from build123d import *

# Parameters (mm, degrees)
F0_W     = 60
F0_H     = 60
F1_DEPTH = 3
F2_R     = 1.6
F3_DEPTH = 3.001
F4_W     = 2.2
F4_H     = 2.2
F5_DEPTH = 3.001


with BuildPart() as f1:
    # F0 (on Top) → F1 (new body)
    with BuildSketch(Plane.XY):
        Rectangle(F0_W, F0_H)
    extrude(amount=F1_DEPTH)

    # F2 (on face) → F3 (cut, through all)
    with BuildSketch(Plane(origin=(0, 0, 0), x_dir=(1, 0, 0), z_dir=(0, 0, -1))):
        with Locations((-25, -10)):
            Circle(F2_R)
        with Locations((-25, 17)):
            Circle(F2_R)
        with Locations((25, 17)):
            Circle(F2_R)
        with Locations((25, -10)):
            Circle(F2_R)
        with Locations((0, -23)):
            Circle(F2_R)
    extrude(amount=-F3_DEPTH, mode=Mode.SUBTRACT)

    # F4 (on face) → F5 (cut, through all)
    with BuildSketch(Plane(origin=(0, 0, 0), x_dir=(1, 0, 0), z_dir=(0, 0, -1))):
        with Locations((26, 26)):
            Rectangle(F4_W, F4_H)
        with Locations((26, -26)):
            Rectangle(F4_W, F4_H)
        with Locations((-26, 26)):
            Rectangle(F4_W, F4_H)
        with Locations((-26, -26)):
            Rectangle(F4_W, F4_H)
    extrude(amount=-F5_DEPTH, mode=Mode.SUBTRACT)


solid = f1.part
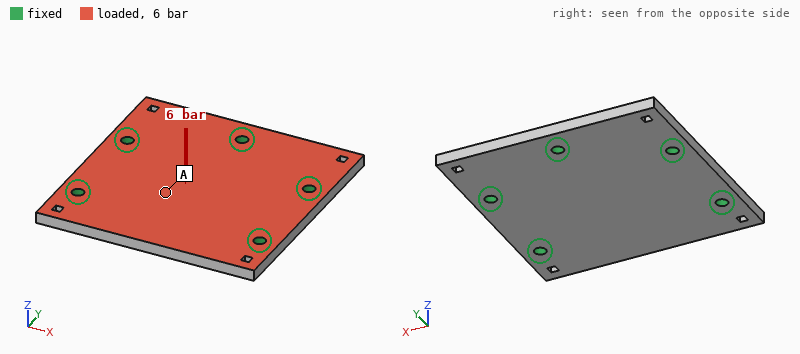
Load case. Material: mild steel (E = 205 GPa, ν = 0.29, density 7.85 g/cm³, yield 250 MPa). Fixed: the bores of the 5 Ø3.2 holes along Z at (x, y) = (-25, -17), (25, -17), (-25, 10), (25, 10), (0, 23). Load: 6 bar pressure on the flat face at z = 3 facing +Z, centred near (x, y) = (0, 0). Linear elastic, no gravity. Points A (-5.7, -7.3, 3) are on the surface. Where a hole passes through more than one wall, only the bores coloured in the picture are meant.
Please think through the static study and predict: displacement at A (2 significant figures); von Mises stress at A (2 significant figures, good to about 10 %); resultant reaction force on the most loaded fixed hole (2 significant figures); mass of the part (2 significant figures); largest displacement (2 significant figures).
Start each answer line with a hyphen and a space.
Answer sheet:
- 19 µm
- 29 MPa
- 480 N
- 83 g
- 35 µm
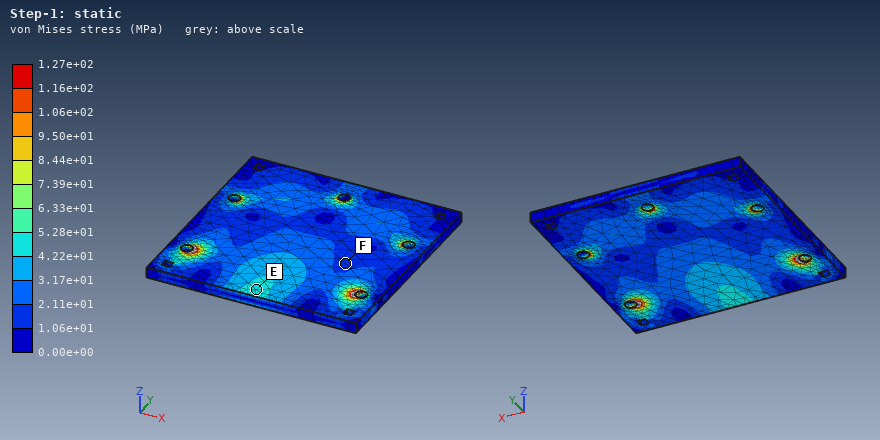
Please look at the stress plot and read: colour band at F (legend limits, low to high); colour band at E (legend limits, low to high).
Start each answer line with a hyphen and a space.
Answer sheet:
- 1.06e+01 to 2.11e+01 MPa
- 4.22e+01 to 5.28e+01 MPa
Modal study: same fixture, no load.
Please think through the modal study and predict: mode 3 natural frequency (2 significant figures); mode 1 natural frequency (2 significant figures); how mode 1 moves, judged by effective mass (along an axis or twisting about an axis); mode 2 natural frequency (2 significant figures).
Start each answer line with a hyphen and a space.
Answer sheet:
- 8700 Hz
- 5700 Hz
- along Z
- 8200 Hz
